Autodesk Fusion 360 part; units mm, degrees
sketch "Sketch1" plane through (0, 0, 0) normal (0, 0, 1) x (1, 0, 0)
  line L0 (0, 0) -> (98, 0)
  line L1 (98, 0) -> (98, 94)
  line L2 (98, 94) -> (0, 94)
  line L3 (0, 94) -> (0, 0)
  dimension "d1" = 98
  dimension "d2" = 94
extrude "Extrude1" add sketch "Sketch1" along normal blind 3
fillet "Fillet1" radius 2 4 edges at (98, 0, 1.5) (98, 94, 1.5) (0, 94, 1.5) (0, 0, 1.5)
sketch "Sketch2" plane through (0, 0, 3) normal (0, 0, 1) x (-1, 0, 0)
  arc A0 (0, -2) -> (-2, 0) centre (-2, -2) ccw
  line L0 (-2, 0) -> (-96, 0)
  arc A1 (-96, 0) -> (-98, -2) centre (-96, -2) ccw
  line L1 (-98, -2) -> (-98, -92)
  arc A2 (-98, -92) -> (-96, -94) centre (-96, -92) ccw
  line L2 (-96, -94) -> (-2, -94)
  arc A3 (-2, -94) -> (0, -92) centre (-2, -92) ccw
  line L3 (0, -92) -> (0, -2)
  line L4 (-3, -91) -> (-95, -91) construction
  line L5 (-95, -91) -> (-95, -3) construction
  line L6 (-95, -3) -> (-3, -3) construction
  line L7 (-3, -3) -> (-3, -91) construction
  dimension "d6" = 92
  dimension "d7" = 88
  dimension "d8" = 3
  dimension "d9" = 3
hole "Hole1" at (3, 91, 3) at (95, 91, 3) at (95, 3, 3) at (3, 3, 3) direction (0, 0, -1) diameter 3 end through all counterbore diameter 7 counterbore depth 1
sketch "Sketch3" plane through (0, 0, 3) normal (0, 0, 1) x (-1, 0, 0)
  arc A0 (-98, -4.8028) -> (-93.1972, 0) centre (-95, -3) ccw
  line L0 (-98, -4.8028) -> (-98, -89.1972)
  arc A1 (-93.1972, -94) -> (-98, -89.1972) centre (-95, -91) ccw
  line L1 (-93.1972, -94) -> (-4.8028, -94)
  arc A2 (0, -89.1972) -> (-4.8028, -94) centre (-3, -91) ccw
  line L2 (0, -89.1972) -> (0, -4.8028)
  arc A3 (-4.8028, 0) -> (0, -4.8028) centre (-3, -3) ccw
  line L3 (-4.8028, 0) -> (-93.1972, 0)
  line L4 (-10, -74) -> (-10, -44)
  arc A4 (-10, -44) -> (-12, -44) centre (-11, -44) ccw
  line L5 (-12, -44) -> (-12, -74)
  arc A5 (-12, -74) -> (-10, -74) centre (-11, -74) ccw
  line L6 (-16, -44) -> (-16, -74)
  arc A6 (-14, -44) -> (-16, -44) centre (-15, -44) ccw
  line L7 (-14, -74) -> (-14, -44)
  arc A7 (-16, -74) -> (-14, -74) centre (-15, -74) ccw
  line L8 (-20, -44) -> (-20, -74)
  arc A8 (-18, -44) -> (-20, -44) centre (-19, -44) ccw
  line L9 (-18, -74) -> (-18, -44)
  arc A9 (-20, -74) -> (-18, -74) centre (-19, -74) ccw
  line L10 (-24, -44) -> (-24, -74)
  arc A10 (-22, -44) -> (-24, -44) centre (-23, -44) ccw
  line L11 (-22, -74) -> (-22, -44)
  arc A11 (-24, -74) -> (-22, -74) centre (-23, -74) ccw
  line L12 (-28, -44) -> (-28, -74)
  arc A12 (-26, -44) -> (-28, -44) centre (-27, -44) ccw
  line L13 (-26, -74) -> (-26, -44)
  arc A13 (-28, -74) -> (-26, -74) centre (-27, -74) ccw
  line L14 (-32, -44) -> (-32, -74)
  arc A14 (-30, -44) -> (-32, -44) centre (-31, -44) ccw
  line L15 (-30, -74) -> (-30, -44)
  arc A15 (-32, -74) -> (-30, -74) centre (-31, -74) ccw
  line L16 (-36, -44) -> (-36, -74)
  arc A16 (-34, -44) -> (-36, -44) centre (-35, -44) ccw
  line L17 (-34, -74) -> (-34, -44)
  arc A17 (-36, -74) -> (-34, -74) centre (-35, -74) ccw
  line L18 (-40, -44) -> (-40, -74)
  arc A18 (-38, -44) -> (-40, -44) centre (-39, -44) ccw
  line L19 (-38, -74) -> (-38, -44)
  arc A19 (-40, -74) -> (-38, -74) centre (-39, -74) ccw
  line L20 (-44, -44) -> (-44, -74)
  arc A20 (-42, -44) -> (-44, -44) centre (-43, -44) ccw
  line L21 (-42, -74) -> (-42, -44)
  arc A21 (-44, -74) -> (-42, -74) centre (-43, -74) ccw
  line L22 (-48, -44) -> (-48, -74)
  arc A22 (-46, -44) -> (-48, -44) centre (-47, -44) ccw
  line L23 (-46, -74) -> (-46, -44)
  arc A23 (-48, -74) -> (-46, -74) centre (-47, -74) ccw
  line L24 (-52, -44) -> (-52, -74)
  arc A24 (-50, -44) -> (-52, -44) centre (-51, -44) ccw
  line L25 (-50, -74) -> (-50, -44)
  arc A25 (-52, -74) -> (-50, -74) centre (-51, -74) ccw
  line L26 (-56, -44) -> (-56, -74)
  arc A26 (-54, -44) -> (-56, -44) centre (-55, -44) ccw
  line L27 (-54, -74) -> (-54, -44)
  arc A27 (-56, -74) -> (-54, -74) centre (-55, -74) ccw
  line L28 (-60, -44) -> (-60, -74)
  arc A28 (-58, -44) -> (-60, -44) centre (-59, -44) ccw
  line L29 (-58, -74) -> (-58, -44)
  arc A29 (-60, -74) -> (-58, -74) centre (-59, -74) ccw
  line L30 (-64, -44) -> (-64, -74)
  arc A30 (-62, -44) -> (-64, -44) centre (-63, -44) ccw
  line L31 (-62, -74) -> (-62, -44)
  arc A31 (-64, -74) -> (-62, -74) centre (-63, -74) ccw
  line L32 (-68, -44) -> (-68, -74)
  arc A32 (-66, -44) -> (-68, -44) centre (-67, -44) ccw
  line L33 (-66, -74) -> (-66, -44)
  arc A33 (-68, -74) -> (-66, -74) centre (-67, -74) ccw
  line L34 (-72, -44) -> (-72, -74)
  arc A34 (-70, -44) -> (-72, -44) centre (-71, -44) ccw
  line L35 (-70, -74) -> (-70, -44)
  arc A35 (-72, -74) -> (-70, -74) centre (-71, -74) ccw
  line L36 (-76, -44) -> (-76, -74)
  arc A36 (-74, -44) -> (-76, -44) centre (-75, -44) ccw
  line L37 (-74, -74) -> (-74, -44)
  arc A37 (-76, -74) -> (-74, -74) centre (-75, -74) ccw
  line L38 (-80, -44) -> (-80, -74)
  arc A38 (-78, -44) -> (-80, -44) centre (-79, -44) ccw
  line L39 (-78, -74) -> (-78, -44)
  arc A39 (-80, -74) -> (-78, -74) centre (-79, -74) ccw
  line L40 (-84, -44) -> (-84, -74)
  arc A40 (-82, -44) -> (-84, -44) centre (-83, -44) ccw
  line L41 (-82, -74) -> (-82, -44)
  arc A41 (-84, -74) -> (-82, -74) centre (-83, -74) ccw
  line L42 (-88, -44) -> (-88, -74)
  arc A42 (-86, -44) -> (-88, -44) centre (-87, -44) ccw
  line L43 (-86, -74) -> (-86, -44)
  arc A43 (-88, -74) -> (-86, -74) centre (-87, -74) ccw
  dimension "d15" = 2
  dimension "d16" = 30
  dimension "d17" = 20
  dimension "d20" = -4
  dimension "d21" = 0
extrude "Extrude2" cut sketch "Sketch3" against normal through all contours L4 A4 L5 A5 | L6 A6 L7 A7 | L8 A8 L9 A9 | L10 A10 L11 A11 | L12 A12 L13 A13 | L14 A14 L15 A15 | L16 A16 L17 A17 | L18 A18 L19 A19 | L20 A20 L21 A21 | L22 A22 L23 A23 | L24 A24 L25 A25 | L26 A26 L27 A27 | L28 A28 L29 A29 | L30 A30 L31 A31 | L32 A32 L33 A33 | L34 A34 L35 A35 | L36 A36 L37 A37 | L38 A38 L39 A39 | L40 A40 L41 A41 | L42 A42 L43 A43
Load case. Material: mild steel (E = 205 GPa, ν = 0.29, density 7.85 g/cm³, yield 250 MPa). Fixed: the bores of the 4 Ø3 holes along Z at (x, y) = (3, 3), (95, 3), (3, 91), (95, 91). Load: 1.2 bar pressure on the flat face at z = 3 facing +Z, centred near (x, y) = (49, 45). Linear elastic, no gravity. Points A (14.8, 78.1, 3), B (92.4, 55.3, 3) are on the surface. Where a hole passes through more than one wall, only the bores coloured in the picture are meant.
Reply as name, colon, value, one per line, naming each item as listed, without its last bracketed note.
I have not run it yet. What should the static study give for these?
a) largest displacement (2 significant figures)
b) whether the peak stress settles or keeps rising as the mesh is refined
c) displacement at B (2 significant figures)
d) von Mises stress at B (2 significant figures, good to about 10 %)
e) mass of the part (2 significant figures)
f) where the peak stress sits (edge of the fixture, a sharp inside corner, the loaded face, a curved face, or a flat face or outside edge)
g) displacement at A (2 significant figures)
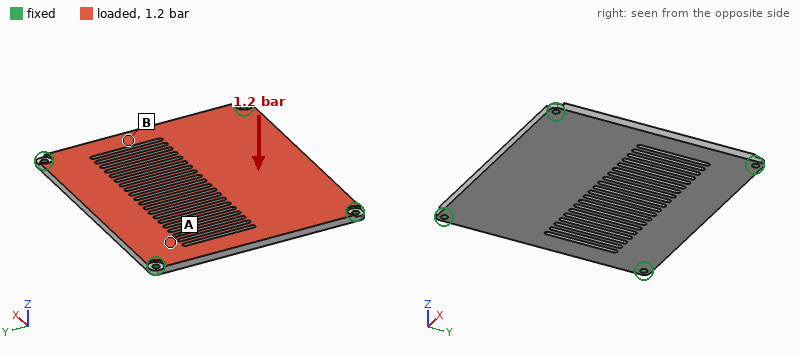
largest displacement: 0.22 mm
whether the peak stress settles or keeps rising as the mesh is refined: keeps rising
displacement at B: 0.100 mm
von Mises stress at B: 51 MPa
mass of the part: 190 g
where the peak stress sits: edge of the fixture
displacement at A: 0.076 mm
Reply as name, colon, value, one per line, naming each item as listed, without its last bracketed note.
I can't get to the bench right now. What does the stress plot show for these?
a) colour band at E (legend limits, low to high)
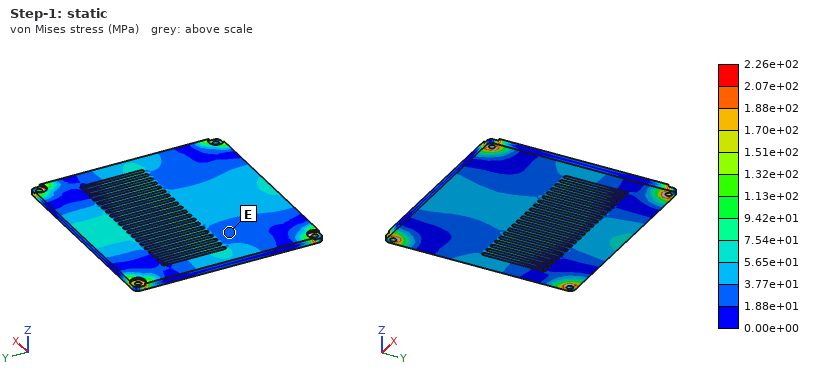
colour band at E: 1.88e+01 to 3.77e+01 MPa
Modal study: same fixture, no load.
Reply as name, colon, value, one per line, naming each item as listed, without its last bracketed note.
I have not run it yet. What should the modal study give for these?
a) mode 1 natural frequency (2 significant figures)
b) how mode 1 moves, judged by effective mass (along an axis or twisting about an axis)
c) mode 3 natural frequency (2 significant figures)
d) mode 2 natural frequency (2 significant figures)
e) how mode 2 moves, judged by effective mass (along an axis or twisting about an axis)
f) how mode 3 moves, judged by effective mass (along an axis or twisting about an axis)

mode 1 natural frequency: 950 Hz
how mode 1 moves, judged by effective mass: along Z
mode 3 natural frequency: 1900 Hz
mode 2 natural frequency: 1700 Hz
how mode 2 moves, judged by effective mass: twisting about X
how mode 3 moves, judged by effective mass: twisting about Y
